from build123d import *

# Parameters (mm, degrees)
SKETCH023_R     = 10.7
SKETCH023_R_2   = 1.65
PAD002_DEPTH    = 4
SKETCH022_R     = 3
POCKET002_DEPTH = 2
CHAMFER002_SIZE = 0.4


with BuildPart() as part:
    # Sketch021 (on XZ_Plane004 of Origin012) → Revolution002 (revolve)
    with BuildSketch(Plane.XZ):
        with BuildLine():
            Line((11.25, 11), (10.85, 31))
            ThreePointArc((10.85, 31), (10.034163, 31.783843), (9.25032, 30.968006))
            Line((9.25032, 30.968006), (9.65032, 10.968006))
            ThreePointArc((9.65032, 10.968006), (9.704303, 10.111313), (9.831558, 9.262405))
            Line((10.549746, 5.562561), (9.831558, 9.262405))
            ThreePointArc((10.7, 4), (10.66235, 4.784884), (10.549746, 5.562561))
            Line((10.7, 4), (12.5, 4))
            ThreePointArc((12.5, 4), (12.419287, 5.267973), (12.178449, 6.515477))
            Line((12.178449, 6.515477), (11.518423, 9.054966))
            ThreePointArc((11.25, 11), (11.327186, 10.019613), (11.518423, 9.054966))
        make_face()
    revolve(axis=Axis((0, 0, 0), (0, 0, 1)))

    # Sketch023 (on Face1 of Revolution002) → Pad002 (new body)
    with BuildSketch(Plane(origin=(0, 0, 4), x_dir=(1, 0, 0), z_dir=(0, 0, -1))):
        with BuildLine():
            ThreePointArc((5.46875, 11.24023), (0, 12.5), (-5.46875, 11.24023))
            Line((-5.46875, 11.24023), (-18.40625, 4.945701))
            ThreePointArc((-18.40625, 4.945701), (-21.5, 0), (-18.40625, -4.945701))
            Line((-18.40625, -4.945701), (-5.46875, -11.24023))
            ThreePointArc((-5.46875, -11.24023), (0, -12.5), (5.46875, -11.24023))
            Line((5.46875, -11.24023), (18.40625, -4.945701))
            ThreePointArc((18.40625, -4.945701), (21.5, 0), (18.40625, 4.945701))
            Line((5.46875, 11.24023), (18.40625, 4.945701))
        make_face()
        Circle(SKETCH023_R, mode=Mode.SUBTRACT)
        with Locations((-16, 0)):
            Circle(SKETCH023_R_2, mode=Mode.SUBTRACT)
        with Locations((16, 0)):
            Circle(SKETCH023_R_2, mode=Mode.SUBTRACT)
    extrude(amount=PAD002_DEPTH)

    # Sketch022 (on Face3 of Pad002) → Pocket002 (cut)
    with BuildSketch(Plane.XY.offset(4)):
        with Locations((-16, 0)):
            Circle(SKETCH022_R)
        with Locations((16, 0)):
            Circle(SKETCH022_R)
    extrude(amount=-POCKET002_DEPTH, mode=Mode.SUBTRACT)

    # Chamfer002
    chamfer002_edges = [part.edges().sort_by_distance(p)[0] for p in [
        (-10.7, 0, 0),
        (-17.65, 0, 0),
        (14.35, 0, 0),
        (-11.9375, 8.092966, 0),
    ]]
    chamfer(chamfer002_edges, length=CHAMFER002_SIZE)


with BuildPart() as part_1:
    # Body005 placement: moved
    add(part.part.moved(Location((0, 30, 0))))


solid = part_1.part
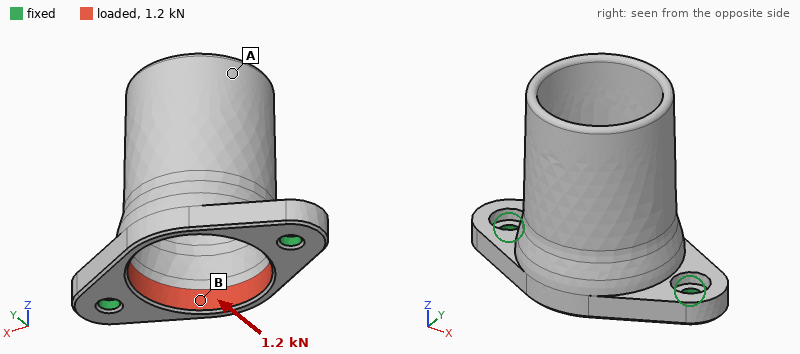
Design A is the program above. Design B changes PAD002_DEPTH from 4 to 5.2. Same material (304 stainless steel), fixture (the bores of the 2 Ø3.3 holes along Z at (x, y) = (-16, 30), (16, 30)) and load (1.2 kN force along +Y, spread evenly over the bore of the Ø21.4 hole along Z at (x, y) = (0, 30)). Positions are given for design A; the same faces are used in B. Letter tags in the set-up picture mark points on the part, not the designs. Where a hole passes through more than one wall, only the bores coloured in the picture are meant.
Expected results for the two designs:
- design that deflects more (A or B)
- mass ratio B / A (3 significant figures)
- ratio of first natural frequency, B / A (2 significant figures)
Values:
A
1.10
1.4
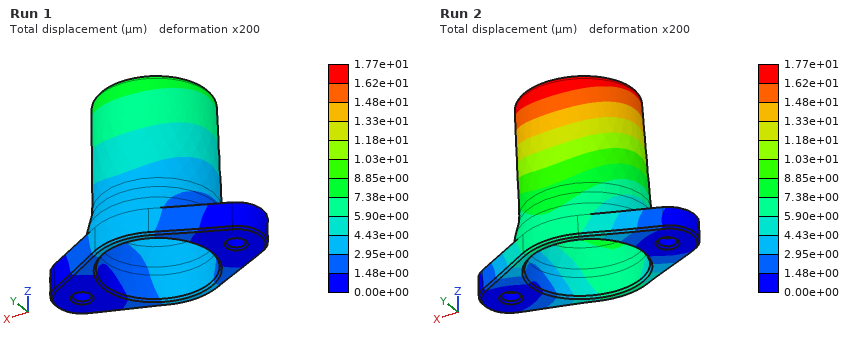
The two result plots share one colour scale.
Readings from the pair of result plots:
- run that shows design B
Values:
Run 1
